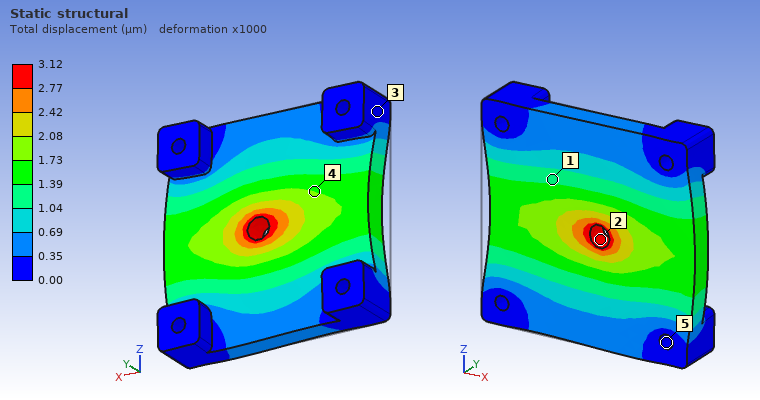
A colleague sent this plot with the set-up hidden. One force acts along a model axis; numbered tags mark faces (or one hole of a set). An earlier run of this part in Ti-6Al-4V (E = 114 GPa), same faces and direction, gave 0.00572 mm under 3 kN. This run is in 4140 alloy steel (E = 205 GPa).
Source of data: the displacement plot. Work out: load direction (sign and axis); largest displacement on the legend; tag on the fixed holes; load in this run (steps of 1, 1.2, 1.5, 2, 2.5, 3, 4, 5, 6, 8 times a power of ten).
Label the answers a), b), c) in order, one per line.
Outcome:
a) +X
b) 3.12 µm
c) 5
d) 3 kN
